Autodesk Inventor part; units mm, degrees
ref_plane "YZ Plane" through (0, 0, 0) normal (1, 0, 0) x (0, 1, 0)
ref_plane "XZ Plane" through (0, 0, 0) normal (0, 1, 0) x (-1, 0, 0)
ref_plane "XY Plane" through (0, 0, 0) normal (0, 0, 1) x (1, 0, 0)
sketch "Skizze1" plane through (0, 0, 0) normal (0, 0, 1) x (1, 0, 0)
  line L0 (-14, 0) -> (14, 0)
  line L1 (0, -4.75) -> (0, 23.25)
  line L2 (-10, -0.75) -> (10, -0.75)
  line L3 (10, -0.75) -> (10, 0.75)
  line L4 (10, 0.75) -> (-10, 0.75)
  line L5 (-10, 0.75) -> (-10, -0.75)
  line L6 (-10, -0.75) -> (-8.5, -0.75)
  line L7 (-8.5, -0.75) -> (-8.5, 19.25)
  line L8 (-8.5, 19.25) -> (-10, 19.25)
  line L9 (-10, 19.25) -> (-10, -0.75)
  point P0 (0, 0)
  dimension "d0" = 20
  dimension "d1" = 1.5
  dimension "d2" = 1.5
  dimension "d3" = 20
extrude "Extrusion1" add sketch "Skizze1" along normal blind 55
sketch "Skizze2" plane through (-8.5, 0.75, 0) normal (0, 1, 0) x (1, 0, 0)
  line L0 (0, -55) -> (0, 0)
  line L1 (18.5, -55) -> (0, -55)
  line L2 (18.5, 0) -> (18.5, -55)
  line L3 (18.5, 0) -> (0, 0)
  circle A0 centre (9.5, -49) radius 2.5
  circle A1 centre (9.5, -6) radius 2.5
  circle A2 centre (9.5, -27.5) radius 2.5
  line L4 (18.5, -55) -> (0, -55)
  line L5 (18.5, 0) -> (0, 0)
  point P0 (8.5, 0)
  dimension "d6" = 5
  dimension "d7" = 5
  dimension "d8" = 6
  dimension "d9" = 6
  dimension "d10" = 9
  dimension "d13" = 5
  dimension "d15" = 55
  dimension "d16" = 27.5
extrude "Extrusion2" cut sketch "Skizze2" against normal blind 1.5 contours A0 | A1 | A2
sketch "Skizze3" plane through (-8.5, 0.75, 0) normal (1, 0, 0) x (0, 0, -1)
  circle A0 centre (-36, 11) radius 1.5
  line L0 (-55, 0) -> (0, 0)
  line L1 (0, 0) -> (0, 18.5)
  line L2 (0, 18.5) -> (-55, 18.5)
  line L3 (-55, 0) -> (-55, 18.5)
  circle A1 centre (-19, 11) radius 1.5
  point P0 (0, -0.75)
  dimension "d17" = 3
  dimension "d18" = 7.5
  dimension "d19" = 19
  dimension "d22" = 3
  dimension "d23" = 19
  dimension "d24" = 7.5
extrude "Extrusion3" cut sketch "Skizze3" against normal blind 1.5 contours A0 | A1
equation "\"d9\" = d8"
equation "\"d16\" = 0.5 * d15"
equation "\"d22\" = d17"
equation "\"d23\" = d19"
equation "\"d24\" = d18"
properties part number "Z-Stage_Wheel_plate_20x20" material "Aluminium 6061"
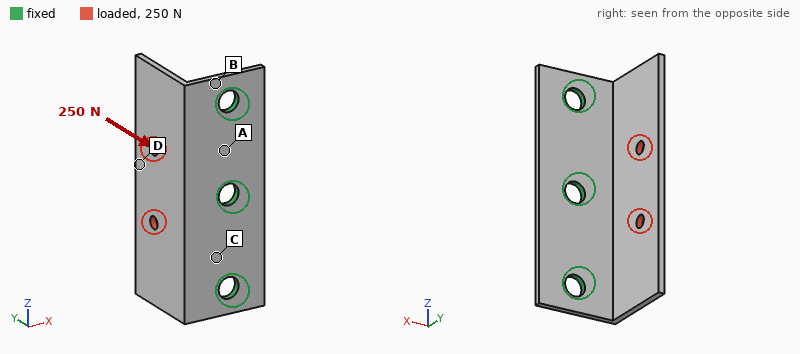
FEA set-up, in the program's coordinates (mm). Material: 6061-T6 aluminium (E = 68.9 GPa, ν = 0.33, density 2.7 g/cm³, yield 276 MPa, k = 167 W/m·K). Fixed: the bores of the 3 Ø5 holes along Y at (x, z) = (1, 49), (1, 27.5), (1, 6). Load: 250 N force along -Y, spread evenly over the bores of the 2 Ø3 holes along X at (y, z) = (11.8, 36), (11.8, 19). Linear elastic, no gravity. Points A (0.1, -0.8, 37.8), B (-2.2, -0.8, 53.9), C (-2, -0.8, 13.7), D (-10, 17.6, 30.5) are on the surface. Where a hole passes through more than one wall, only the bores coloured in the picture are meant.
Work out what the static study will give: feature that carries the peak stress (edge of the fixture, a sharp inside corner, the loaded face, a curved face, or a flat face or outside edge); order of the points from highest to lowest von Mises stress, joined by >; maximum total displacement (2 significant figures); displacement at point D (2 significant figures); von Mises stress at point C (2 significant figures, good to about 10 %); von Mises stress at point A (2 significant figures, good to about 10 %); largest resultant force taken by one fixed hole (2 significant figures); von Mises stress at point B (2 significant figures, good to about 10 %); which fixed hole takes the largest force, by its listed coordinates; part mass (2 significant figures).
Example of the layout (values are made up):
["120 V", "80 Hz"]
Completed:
["a flat face or outside edge", "B > C > A > D", "0.18 mm", "0.17 mm", "43 MPa", "31 MPa", "99 N", "70 MPa", "(1, 27.5)", "8.3 g"]
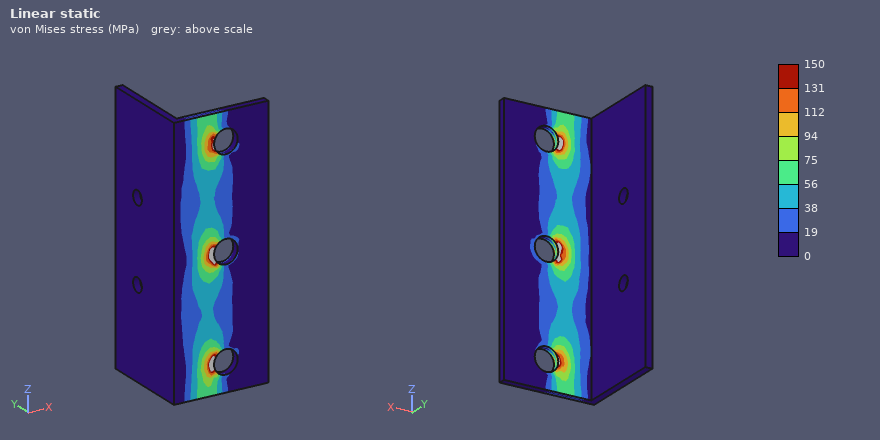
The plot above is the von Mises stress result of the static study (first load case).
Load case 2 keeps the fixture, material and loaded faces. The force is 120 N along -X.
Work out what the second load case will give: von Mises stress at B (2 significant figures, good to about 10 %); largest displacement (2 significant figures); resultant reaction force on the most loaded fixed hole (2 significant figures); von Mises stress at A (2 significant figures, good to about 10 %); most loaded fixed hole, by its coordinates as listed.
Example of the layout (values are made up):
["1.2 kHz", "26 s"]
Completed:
["59 MPa", "0.34 mm", "90 N", "25 MPa", "(1, 27.5)"]
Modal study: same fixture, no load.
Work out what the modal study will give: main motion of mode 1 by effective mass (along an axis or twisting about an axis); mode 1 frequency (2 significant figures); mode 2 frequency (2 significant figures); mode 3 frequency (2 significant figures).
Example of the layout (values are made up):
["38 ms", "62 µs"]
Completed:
["along X", "2000 Hz", "3000 Hz", "6300 Hz"]
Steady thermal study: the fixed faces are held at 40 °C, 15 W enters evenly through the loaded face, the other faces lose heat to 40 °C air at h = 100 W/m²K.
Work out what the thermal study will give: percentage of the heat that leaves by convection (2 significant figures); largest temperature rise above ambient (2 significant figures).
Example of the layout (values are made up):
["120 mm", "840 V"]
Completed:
["27 %", "27 K"]
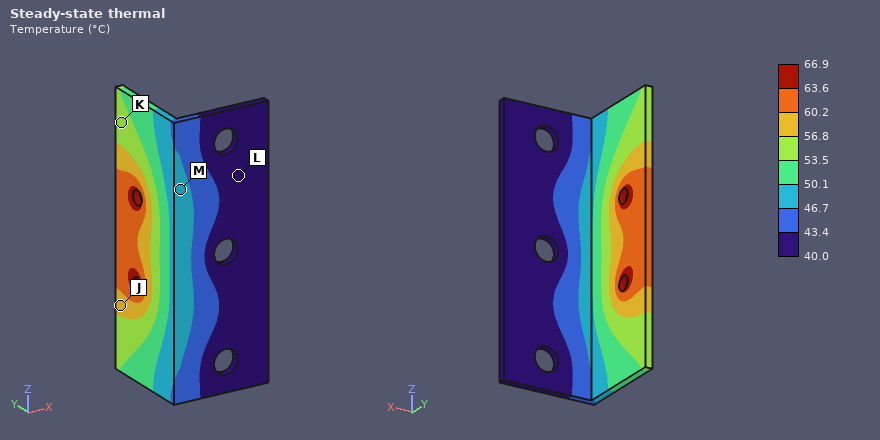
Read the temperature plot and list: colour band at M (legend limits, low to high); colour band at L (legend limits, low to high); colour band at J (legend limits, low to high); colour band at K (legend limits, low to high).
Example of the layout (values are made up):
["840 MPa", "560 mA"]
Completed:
["46.7 to 50.1 °C", "40.0 to 43.4 °C", "56.8 to 60.2 °C", "53.5 to 56.8 °C"]
